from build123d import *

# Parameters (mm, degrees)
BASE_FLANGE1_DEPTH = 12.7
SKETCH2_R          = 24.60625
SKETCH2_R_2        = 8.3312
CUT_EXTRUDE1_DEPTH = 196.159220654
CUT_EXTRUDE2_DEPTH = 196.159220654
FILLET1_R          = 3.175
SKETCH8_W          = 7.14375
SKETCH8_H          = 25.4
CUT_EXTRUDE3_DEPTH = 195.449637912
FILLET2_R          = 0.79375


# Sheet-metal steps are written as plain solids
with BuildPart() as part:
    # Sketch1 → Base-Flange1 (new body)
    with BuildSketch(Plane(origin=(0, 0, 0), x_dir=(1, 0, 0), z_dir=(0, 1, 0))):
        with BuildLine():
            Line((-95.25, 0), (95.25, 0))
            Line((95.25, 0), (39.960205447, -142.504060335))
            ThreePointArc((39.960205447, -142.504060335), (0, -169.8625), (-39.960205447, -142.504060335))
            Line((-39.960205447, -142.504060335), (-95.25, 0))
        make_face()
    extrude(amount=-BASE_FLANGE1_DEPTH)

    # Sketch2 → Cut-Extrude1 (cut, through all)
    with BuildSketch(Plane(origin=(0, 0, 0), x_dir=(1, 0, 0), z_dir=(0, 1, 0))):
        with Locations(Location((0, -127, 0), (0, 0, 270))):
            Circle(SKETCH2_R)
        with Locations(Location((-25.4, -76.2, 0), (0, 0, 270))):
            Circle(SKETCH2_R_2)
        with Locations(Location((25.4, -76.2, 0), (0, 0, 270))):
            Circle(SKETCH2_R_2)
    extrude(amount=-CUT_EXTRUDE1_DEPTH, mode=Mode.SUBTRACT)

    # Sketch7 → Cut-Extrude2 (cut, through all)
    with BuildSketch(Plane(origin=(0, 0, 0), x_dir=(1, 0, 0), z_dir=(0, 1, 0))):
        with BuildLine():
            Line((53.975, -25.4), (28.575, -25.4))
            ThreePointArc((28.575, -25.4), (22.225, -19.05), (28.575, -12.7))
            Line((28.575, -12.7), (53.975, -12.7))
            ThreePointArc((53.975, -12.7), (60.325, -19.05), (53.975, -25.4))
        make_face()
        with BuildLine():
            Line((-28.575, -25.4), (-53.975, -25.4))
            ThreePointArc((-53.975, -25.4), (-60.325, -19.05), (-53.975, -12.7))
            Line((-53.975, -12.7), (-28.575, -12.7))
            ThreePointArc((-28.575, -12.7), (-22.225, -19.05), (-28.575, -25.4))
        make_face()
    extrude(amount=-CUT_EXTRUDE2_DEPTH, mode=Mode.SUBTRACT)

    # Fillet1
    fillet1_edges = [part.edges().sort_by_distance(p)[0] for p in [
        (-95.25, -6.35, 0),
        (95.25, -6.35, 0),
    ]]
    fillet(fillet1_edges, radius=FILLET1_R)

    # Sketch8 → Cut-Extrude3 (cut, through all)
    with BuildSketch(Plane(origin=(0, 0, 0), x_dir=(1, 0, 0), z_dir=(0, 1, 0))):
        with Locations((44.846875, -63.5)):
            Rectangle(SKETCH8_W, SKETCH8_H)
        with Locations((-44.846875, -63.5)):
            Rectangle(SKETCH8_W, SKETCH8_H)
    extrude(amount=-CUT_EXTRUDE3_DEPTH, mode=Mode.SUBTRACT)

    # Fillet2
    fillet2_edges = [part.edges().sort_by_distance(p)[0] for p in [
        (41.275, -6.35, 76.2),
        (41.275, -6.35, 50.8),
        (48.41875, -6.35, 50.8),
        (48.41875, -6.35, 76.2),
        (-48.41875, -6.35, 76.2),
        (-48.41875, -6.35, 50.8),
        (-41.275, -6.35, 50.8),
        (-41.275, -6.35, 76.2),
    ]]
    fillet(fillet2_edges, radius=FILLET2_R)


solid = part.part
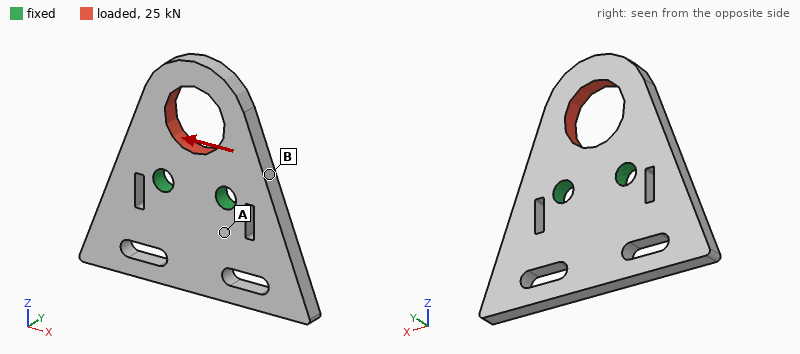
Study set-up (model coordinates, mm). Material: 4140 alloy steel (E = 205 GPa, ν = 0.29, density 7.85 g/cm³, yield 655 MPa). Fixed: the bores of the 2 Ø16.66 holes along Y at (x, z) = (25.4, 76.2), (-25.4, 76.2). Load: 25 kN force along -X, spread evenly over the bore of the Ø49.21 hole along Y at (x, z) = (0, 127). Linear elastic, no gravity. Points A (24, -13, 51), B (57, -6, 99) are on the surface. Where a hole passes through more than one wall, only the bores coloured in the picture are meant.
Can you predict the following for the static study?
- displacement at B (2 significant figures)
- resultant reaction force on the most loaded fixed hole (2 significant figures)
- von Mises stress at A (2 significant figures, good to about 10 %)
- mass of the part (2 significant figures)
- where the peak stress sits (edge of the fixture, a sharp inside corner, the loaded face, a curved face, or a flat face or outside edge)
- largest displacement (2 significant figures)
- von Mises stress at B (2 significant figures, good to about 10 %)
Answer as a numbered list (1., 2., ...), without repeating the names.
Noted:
1. 19 µm
2. 21 kN
3. 12 MPa
4. 1.7 kg
5. a curved face
6. 63 µm
7. 52 MPa
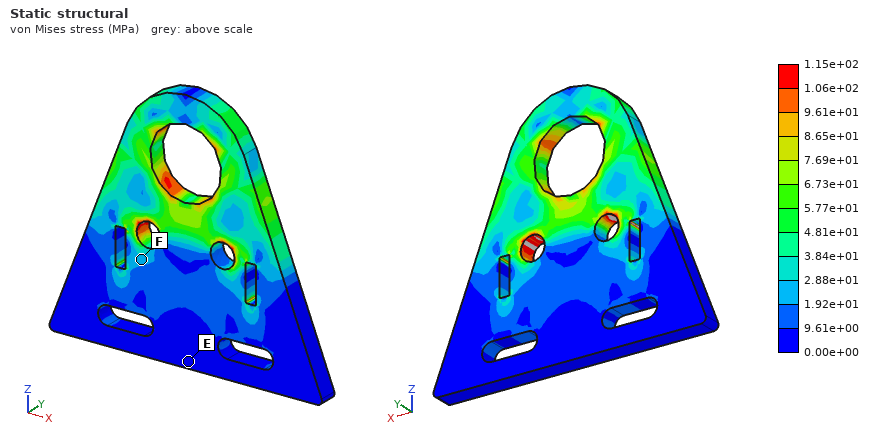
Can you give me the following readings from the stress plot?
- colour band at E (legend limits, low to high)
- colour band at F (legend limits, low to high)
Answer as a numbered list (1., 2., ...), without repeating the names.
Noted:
1. 0.00e+00 to 9.61e+00 MPa
2. 1.92e+01 to 2.88e+01 MPa
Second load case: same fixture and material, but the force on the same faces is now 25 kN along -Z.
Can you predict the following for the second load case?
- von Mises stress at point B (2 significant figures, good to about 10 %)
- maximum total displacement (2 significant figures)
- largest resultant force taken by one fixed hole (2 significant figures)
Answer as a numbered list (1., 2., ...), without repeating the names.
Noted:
1. 11 MPa
2. 18 µm
3. 13 kN
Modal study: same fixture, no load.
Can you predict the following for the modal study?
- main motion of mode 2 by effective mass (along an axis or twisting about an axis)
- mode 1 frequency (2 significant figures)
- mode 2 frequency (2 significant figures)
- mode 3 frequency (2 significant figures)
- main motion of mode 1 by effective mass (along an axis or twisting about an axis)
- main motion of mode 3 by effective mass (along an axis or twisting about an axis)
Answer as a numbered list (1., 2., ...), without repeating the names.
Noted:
1. twisting about Z
2. 1500 Hz
3. 1600 Hz
4. 1700 Hz
5. along Y
6. along Y
